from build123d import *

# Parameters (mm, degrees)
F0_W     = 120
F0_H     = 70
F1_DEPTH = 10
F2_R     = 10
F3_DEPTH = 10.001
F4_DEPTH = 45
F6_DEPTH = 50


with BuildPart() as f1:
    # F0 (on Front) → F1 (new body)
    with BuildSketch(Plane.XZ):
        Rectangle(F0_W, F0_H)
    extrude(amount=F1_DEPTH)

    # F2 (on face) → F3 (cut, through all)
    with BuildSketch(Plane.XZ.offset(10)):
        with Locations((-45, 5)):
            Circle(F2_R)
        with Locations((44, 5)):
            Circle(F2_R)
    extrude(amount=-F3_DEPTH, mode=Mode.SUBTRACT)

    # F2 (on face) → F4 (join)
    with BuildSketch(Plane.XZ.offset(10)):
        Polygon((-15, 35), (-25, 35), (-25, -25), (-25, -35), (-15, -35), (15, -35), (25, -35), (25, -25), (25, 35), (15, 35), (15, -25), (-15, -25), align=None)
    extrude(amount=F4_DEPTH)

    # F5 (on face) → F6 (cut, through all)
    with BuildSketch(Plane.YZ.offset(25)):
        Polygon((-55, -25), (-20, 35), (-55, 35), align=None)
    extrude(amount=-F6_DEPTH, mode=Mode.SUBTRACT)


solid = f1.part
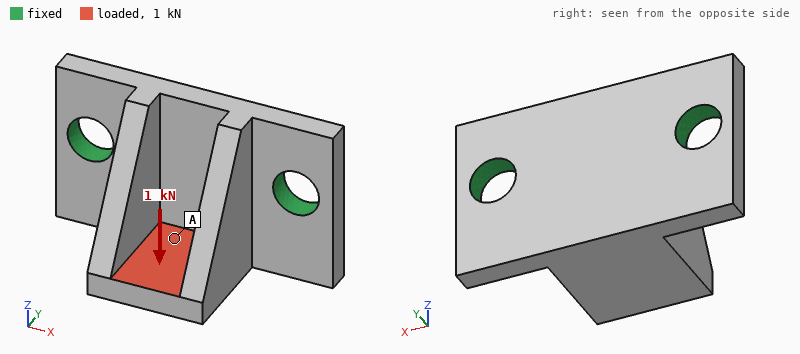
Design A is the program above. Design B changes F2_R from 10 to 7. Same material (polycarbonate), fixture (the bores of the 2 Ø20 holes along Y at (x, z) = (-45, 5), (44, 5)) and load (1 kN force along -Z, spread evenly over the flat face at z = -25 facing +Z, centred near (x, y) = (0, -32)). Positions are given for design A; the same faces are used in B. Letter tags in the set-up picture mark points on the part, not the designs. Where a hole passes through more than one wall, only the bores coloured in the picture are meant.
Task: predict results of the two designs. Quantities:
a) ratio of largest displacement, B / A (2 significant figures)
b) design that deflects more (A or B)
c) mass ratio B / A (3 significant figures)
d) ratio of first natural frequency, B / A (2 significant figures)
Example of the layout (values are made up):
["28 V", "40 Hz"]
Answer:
["1.4", "B", "1.02", "0.83"]
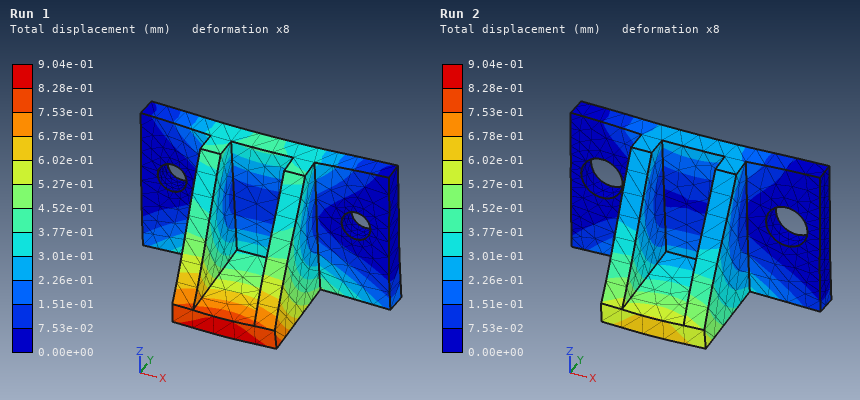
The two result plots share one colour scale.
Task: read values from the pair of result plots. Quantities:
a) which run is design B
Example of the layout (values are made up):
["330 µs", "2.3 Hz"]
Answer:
["Run 1"]
